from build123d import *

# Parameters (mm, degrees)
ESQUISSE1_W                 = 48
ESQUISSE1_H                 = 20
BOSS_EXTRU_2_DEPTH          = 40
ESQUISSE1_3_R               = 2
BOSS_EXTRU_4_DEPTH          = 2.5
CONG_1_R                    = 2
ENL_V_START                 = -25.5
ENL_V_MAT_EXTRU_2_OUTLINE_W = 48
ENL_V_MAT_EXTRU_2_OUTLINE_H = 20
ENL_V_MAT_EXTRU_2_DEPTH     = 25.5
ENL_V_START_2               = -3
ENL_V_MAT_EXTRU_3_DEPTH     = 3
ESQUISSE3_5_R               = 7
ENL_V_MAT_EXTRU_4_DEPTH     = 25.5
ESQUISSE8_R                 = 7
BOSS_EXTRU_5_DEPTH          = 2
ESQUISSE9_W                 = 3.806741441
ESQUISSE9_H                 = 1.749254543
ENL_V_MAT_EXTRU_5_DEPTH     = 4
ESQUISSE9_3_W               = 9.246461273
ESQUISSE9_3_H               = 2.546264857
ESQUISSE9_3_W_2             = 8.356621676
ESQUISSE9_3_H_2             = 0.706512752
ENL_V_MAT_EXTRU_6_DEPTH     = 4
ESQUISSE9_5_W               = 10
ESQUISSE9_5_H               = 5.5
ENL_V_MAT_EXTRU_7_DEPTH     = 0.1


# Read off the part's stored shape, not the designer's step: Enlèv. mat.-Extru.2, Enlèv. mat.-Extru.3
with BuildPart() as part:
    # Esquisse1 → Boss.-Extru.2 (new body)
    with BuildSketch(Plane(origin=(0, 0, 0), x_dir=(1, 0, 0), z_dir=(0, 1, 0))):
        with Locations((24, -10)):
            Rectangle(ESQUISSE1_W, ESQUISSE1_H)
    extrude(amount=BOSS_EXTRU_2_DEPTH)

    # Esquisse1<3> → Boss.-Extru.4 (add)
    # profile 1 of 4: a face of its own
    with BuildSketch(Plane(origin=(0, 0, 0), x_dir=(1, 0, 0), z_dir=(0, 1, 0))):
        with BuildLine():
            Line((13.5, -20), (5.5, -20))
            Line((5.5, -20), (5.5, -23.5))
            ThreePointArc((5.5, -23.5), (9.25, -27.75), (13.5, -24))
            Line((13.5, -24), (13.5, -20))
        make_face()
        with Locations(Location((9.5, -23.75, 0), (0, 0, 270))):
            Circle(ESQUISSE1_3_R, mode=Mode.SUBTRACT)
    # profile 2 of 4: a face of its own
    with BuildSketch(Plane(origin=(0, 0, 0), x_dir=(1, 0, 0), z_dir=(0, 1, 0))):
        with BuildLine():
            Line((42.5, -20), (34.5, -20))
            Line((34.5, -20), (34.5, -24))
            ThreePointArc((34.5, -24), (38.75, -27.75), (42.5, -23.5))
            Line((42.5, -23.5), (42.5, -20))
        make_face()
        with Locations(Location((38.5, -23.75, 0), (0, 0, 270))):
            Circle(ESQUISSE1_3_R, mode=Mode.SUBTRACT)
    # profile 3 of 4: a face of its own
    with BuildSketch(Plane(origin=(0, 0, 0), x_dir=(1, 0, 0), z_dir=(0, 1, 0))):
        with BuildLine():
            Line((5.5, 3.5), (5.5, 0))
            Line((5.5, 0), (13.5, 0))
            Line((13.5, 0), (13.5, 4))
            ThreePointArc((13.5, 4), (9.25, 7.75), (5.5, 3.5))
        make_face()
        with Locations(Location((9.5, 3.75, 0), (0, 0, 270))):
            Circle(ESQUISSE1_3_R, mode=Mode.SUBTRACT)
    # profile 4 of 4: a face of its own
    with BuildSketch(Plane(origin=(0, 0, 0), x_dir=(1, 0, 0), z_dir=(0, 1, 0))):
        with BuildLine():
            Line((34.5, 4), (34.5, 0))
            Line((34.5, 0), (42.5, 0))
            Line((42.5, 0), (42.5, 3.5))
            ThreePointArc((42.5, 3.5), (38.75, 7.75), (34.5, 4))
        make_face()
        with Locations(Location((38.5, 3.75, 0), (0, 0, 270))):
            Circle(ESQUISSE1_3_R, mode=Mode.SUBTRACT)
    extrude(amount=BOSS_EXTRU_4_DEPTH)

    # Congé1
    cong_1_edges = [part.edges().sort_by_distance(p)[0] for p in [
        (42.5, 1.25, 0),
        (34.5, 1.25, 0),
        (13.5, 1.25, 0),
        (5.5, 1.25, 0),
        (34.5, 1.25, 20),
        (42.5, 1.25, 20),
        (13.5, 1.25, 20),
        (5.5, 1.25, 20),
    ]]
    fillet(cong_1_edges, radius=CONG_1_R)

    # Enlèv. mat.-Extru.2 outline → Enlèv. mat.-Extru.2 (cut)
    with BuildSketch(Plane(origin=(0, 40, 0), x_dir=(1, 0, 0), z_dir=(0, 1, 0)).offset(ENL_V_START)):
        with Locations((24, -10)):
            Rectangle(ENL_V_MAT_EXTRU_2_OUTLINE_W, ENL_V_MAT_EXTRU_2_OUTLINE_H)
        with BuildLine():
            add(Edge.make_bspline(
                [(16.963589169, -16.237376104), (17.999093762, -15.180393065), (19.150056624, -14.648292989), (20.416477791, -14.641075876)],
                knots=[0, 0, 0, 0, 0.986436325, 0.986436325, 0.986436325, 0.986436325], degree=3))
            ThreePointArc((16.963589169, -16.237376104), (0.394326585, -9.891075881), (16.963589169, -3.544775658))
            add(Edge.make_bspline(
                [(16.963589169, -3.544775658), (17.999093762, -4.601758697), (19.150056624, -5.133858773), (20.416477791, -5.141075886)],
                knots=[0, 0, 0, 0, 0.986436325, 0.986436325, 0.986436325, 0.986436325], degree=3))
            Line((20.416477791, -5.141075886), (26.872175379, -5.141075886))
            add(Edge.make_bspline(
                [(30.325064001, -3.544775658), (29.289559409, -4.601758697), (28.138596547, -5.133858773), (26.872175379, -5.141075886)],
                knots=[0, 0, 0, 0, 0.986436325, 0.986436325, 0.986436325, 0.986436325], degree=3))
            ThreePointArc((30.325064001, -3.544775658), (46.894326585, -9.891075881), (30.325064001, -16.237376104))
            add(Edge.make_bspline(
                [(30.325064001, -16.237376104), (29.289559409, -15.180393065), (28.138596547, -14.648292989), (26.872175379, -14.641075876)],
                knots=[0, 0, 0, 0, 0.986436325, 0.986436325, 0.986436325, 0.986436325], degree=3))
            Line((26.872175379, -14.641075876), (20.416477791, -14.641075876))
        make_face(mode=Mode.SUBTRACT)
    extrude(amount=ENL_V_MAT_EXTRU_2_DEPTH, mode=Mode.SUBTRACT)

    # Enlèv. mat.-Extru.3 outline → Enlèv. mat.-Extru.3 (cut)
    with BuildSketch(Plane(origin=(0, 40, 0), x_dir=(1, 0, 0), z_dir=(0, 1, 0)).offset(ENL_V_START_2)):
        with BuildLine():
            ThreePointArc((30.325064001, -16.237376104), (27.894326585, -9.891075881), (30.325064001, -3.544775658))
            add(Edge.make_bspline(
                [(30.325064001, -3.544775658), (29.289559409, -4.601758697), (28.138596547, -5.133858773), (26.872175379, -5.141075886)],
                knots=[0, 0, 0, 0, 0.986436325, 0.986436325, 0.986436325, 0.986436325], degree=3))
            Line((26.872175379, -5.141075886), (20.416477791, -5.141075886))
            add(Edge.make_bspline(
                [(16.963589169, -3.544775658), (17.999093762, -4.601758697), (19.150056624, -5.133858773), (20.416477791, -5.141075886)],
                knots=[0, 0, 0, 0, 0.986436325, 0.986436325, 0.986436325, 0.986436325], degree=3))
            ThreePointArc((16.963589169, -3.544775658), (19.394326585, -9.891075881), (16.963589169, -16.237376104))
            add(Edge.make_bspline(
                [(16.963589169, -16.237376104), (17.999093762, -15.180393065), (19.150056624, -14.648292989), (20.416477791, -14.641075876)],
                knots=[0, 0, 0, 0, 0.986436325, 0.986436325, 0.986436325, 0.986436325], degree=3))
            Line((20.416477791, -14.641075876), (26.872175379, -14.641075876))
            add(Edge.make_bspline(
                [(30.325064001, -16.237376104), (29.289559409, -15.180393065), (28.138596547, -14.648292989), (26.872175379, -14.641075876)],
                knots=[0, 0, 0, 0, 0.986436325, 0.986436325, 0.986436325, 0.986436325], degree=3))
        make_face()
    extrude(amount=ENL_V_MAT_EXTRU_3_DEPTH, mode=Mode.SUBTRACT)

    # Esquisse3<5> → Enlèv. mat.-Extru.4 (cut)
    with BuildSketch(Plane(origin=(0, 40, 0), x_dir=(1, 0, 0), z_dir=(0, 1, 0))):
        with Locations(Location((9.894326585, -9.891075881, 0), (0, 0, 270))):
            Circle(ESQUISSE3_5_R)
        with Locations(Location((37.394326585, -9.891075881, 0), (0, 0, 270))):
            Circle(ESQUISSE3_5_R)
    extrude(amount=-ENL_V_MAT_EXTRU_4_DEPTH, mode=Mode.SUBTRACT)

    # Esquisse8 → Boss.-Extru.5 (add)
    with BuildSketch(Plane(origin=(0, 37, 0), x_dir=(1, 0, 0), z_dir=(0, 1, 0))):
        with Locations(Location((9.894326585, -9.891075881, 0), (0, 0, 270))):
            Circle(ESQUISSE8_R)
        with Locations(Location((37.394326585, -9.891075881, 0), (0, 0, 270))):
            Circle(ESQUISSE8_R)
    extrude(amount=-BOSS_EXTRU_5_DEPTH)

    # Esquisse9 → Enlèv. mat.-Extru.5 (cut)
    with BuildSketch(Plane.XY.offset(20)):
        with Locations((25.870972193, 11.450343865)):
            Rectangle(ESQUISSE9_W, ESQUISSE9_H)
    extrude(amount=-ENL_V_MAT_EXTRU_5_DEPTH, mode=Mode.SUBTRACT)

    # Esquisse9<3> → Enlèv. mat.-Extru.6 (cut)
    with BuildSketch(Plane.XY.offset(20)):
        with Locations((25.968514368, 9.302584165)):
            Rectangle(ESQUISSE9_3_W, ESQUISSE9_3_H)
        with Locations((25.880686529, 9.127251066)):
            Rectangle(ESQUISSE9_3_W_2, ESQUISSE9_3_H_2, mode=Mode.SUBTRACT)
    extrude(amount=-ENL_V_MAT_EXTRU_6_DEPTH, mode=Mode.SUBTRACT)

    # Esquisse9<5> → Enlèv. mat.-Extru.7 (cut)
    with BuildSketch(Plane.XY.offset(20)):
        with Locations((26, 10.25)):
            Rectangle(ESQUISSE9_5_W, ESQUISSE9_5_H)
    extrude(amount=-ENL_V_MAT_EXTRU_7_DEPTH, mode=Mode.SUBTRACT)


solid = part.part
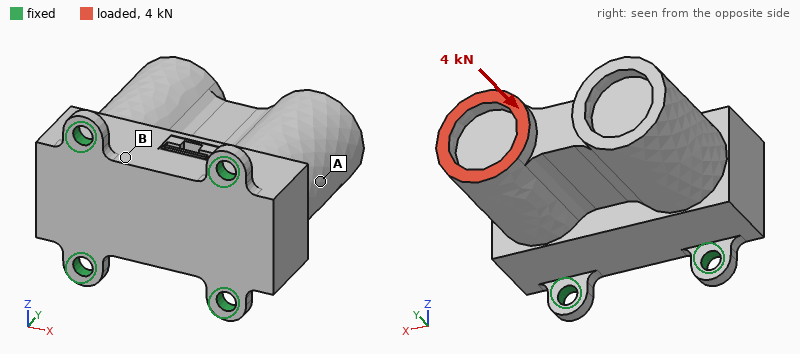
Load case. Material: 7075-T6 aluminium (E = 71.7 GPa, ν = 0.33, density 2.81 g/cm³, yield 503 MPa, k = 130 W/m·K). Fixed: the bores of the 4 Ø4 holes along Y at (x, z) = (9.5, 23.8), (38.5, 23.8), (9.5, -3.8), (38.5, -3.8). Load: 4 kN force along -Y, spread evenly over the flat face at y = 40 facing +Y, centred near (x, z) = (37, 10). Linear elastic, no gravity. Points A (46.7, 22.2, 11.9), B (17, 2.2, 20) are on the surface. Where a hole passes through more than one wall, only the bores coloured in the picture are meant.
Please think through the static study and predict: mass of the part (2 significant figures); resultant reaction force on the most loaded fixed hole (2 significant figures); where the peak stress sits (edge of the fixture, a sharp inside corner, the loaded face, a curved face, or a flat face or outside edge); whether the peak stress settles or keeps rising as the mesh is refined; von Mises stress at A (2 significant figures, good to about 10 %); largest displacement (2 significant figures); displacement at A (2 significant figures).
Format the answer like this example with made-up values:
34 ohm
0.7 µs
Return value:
66 g
2.1 kN
edge of the fixture
keeps rising
33 MPa
60 µm
43 µm
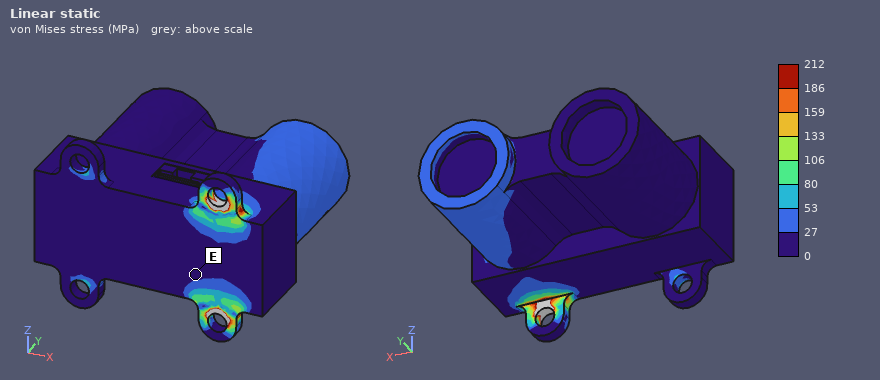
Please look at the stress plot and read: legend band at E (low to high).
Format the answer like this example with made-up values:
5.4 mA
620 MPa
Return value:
0 to 27 MPa
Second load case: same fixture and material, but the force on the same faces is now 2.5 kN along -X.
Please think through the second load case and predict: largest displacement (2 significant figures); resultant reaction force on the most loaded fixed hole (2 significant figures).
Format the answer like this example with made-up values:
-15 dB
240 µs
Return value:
0.11 mm
1.9 kN
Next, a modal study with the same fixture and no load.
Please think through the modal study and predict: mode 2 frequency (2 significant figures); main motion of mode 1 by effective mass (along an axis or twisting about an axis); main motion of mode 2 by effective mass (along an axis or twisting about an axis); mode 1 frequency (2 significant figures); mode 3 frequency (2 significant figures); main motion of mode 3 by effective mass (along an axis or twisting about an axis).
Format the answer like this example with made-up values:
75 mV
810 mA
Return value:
6200 Hz
along Z
along X
5600 Hz
11 kHz
along Y
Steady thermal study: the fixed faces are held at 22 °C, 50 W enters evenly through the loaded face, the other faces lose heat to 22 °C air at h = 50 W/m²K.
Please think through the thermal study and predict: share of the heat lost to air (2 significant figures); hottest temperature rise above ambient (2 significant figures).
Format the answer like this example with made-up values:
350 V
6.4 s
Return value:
26 %
72 K
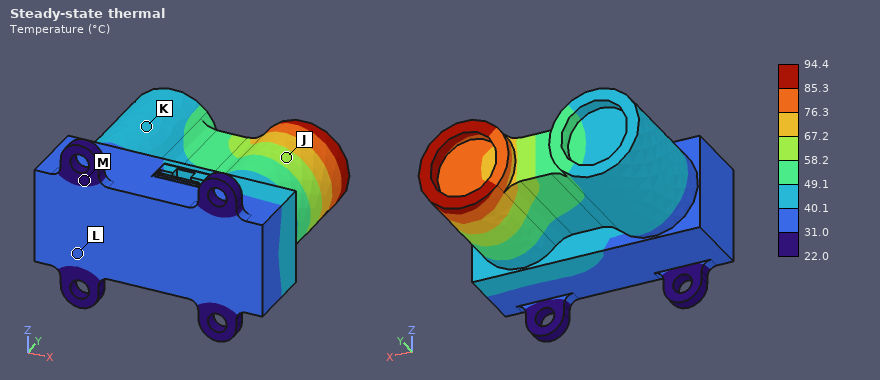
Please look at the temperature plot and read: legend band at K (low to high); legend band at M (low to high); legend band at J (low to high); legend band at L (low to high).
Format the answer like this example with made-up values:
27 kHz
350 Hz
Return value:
40.1 to 49.1 °C
22.0 to 31.0 °C
58.2 to 67.2 °C
31.0 to 40.1 °C
